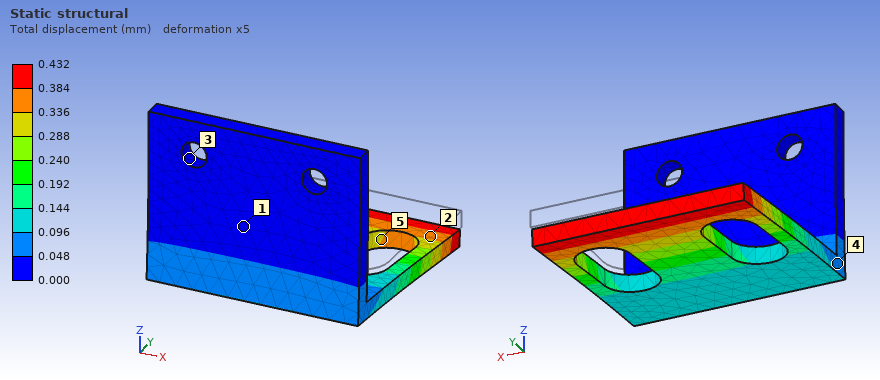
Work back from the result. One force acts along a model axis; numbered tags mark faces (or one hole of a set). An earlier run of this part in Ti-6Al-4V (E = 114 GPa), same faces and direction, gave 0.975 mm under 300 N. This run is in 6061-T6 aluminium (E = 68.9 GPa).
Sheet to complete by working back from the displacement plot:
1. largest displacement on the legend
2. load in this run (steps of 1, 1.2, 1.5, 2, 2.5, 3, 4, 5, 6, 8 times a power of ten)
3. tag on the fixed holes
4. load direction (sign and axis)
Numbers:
0.432 mm
80 N
3
-Z
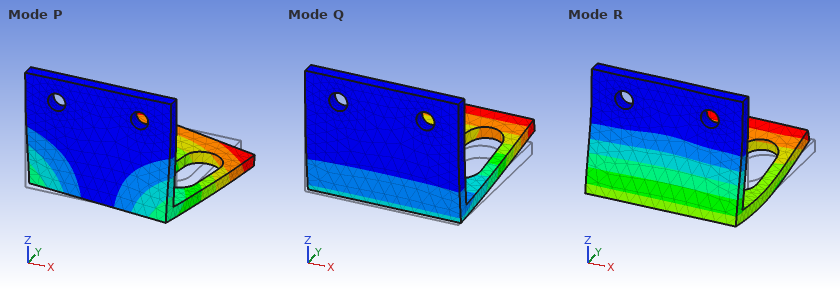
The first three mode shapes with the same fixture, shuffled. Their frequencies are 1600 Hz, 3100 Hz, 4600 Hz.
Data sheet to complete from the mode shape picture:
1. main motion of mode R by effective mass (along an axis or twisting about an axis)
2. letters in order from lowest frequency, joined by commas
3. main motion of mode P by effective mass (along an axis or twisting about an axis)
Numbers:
along Y
Q, P, R
along X
